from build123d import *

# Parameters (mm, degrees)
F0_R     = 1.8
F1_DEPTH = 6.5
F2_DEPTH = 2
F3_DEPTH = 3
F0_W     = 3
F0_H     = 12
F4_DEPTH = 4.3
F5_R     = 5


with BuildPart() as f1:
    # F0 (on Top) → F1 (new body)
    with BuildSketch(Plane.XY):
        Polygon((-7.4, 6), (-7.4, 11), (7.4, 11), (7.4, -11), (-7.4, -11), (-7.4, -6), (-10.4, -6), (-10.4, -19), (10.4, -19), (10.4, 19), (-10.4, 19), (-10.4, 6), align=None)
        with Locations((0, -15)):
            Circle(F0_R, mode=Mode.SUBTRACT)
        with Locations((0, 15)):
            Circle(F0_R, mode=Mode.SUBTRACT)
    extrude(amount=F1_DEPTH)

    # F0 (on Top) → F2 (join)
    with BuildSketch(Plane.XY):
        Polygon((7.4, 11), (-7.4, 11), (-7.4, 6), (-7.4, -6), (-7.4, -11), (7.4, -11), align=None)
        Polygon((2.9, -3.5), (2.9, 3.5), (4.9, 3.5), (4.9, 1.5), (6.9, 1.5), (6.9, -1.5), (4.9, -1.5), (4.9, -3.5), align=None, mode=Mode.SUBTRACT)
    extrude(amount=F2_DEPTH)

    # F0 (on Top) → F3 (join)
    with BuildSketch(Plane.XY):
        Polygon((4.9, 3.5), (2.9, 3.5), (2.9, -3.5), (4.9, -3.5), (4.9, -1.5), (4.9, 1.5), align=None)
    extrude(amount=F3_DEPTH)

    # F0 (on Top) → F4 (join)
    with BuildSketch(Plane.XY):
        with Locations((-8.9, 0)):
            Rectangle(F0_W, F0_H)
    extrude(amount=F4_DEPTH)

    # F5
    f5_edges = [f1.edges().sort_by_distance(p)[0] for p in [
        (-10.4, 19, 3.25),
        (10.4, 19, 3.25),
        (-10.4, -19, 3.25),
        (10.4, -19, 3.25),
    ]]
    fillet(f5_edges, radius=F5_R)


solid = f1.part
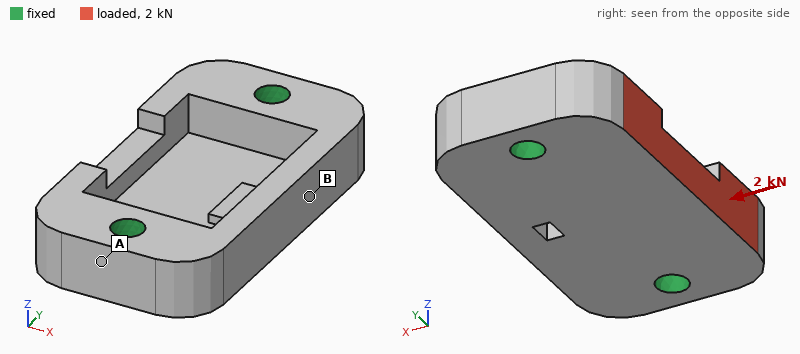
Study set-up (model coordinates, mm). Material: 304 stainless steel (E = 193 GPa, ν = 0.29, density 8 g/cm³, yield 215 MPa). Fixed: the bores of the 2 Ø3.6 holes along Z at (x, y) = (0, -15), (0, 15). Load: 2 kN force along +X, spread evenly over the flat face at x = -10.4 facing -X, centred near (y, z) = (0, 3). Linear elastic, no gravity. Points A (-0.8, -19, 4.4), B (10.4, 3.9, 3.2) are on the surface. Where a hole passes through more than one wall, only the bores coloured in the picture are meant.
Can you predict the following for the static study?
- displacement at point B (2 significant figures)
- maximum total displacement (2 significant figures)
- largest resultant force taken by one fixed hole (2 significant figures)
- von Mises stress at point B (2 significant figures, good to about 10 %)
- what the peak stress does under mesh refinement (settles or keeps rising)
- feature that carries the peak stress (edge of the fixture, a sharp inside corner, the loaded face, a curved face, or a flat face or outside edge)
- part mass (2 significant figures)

1.4 µm
7.1 µm
1.0 kN
15 MPa
keeps rising
a sharp inside corner
27 g
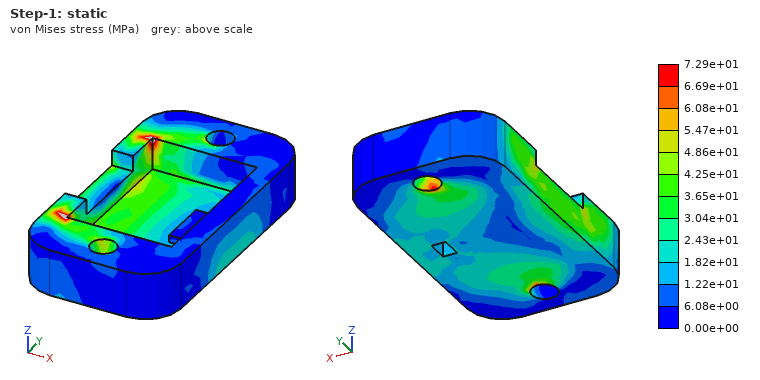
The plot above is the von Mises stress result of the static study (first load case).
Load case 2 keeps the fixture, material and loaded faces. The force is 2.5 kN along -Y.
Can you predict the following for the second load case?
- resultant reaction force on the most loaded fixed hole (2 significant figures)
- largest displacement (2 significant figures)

1.4 kN
6.1 µm
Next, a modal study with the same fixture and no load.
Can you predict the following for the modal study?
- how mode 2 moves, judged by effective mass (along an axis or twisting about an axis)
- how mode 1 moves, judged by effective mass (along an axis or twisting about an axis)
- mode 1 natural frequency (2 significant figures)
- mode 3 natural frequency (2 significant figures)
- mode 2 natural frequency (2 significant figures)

twisting about Y
along Z
20 kHz
32 kHz
22 kHz
